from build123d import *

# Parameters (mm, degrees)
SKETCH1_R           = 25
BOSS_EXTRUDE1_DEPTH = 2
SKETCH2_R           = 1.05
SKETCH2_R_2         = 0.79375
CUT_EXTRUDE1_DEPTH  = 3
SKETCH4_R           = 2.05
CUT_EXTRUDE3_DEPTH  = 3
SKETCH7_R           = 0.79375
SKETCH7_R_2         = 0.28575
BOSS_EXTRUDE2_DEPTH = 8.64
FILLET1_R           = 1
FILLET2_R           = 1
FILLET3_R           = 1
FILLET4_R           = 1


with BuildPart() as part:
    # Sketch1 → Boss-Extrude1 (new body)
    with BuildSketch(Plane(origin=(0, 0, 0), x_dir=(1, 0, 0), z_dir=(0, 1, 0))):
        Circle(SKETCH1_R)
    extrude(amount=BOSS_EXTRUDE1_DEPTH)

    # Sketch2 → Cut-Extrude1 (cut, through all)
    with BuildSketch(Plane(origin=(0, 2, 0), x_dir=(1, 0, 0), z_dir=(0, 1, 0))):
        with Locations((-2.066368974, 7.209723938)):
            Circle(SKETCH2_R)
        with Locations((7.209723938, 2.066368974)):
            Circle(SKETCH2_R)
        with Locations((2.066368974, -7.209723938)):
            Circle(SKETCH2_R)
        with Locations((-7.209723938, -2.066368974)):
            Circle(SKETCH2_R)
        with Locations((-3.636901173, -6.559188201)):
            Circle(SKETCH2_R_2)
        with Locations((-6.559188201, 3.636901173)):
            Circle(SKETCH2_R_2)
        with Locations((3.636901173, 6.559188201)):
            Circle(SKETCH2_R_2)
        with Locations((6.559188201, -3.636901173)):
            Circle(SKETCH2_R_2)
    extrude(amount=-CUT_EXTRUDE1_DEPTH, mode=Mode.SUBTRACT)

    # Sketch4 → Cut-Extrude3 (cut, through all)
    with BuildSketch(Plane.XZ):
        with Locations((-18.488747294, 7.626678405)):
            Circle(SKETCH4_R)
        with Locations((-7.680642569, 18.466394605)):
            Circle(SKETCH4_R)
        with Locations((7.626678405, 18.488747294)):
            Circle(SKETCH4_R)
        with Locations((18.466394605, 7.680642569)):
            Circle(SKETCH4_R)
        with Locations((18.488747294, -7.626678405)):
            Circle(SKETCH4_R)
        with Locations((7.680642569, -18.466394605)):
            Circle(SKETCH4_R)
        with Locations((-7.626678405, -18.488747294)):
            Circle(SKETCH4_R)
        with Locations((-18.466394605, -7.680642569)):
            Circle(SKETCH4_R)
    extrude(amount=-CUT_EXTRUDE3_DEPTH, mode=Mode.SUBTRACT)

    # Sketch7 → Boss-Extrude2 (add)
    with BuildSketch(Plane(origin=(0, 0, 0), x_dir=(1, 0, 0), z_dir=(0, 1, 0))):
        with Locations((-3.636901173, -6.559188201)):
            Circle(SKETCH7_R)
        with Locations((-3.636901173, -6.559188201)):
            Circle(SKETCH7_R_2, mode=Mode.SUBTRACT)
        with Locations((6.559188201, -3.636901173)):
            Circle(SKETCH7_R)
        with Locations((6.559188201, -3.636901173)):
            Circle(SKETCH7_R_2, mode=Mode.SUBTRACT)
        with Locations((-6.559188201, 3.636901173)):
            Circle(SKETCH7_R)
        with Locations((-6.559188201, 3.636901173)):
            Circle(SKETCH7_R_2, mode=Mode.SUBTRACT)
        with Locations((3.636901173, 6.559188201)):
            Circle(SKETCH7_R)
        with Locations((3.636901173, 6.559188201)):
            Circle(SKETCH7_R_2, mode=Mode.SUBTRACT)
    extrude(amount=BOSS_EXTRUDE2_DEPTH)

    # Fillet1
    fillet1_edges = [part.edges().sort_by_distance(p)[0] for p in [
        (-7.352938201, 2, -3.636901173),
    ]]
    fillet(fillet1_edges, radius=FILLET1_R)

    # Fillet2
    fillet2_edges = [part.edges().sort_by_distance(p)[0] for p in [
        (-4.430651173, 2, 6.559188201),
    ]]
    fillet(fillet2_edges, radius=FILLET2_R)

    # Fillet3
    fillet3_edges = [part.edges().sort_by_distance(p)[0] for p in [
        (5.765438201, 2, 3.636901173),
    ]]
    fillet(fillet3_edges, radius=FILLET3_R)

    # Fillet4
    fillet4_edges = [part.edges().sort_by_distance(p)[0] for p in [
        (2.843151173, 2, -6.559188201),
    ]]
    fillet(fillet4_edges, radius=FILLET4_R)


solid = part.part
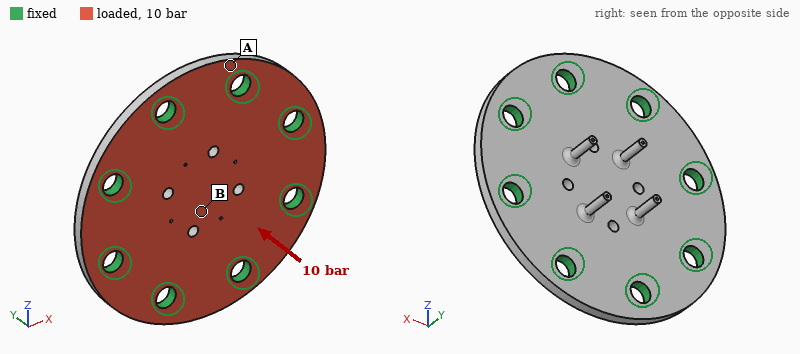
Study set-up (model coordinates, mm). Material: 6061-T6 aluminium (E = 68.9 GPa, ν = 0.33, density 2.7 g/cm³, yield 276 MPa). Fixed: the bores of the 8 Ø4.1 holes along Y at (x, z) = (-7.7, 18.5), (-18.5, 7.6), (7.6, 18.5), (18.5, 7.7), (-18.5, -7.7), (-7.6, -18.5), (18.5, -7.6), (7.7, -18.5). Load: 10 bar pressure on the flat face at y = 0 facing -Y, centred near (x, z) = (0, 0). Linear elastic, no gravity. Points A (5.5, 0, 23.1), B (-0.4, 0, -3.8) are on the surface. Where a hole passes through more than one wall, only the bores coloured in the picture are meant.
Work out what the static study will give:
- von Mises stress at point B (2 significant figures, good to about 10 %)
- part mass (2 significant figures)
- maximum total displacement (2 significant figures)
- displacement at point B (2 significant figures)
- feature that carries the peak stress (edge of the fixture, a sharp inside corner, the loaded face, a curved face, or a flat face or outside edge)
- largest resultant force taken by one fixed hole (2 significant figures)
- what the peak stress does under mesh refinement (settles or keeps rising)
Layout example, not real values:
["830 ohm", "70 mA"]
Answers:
["40 MPa", "10 g", "43 µm", "40 µm", "edge of the fixture", "230 N", "keeps rising"]
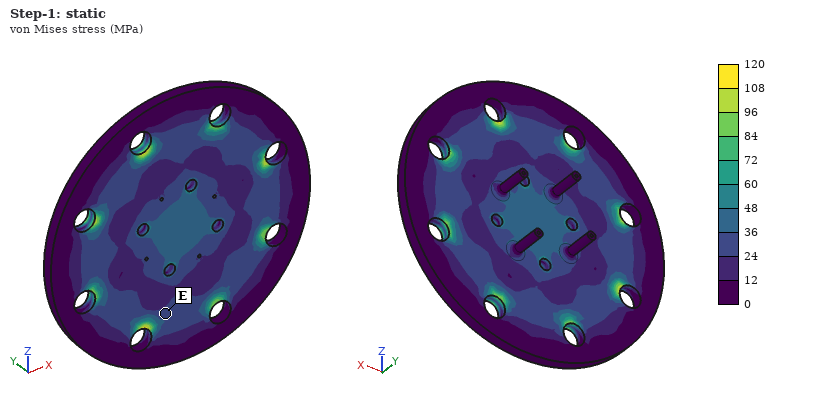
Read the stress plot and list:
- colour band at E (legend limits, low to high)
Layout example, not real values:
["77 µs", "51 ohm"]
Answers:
["24 to 36 MPa"]
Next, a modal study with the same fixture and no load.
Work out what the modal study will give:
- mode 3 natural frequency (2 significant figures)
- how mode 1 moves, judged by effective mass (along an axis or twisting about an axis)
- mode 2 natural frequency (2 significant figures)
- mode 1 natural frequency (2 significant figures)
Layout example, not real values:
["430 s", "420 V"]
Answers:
["24 kHz", "along Y", "24 kHz", "13 kHz"]
